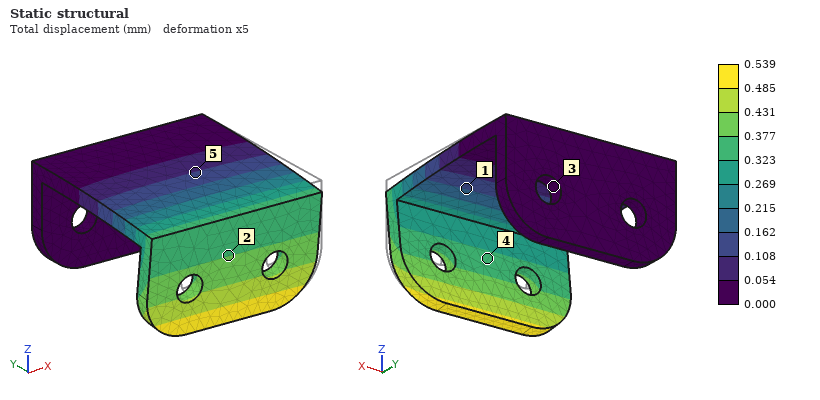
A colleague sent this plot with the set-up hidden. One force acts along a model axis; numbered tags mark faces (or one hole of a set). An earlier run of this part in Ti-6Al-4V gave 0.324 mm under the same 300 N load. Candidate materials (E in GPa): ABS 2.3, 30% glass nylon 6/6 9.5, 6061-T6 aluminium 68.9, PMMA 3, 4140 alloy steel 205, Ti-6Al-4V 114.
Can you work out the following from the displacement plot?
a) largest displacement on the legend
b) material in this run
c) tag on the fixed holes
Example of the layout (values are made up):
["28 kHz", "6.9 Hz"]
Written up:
["0.539 mm", "6061-T6 aluminium", "3"]
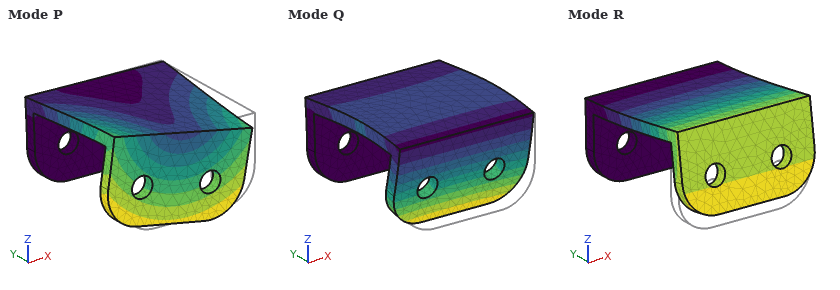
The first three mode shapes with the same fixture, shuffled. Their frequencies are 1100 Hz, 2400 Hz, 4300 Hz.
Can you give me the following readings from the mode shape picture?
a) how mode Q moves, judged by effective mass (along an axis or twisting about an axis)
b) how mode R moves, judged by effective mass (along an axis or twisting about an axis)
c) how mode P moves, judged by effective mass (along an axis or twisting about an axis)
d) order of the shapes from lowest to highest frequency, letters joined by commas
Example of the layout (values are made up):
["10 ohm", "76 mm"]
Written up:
["along Y", "along Z", "along X", "R, P, Q"]
